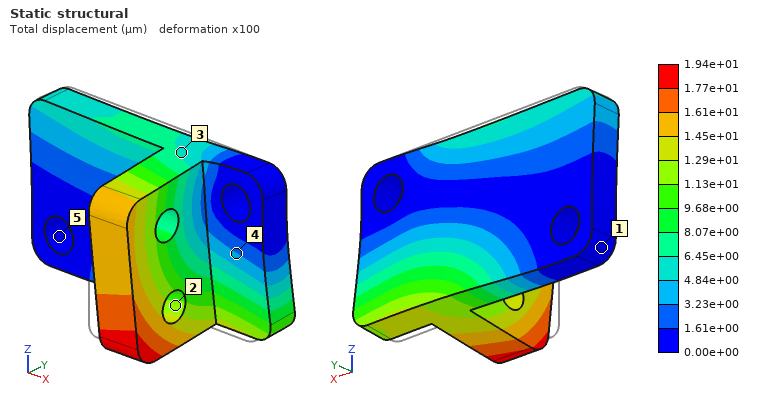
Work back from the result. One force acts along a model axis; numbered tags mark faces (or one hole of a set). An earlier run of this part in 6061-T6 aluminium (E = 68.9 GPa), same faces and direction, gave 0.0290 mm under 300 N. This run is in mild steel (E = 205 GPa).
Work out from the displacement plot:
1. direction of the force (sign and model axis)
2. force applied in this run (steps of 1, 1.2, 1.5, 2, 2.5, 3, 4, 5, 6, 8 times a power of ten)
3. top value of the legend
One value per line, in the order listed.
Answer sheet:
-Z
600 N
1.94e+01 µm
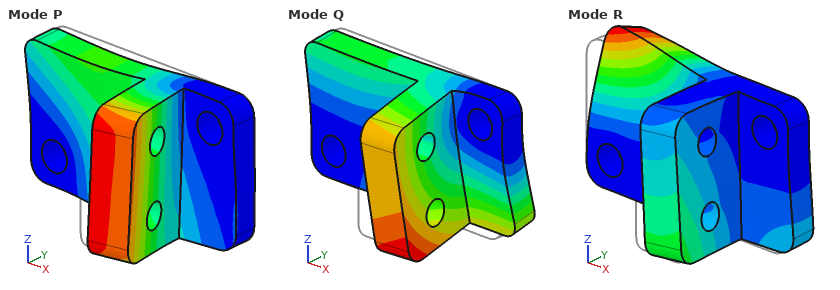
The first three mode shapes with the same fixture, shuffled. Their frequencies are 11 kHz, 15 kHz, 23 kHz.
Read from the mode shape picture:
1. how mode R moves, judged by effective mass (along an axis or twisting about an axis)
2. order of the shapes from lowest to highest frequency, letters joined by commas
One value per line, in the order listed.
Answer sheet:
along Y
Q, P, R
